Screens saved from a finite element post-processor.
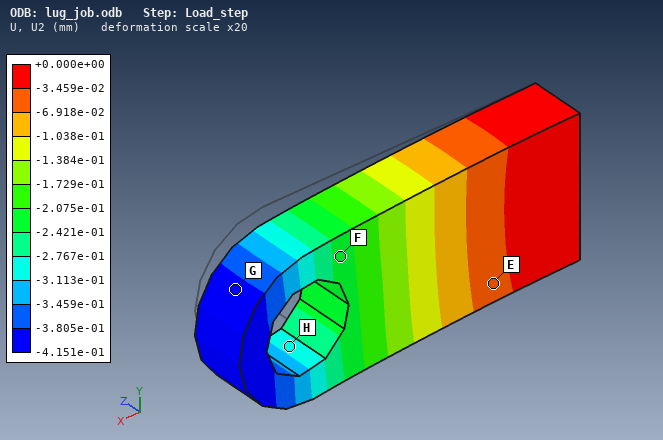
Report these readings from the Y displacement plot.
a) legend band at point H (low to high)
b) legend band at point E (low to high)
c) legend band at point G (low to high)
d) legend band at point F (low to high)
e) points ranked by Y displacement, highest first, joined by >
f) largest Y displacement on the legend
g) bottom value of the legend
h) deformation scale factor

-3.113e-01 to -2.767e-01 mm
-6.918e-02 to -3.459e-02 mm
-4.151e-01 to -3.805e-01 mm
-2.421e-01 to -2.075e-01 mm
E > F > H > G
+0.000e+00 mm
-4.151e-01 mm
20
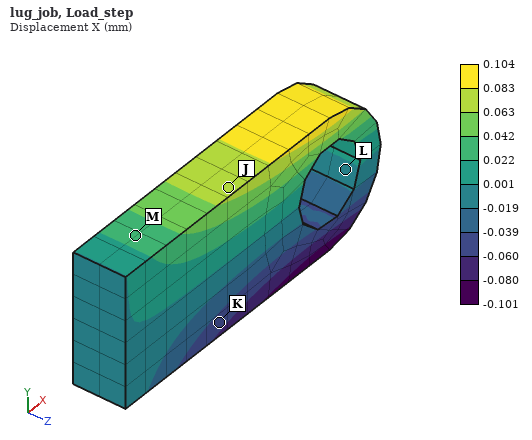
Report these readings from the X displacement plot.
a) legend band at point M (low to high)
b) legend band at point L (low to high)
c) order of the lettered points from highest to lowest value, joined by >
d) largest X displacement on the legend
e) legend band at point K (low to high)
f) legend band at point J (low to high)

0.022 to 0.042 mm
-0.019 to 0.001 mm
J > M > L > K
0.104 mm
-0.060 to -0.039 mm
0.063 to 0.083 mm
